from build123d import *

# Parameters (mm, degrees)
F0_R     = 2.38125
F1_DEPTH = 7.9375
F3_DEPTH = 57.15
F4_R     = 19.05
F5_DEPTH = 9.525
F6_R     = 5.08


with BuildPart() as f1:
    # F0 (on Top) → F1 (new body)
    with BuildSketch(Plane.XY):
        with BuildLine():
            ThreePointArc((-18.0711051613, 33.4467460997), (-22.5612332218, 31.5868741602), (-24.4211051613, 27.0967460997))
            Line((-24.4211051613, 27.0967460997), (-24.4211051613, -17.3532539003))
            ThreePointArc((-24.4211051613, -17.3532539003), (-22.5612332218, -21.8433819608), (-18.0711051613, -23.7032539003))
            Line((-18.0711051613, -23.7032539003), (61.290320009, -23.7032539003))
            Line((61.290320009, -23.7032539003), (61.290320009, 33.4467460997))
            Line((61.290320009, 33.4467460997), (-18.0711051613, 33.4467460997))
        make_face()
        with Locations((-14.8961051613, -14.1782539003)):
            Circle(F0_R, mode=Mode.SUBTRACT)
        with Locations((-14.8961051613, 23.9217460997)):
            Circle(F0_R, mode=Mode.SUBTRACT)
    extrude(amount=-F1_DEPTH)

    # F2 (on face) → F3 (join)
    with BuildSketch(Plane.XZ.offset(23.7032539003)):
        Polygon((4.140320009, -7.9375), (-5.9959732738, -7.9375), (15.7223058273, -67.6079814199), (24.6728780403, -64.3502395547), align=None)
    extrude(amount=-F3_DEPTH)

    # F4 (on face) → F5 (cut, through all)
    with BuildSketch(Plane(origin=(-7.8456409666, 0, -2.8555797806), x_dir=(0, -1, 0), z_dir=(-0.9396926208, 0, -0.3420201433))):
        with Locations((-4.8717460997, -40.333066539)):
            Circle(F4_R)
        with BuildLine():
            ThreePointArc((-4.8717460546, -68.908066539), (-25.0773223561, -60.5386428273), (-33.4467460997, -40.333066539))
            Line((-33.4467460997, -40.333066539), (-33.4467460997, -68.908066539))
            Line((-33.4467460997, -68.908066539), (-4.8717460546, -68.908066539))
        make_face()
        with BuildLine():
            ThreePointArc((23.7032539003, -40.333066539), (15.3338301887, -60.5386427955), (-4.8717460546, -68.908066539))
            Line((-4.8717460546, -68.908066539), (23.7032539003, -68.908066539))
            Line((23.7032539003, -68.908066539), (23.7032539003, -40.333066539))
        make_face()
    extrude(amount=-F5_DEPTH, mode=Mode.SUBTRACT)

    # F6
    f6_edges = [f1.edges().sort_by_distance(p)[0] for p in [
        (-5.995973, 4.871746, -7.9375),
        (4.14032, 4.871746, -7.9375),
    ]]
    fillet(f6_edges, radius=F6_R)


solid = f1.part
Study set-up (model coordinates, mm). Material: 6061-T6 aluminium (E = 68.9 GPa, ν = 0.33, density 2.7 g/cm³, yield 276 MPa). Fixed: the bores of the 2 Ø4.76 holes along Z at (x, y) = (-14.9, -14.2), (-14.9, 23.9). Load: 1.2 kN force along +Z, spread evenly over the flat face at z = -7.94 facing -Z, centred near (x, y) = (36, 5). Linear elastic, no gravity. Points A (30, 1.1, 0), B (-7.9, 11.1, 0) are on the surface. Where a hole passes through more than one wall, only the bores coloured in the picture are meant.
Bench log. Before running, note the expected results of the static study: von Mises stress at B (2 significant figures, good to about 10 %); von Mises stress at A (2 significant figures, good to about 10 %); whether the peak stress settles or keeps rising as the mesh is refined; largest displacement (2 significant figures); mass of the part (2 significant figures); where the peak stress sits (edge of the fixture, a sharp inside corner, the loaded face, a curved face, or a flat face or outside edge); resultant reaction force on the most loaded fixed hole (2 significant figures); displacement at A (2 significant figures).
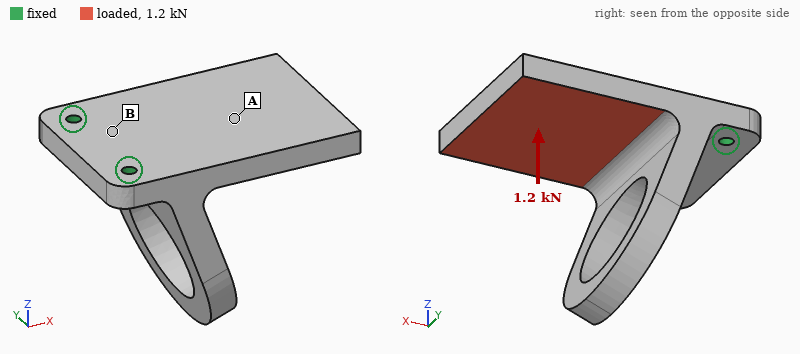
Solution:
53 MPa
18 MPa
keeps rising
0.51 mm
160 g
edge of the fixture
610 N
0.24 mm
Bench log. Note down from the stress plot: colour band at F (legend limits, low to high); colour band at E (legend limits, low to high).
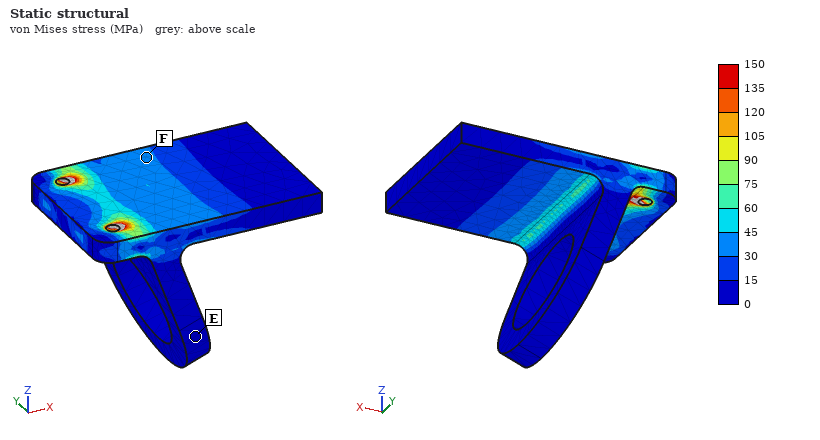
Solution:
30 to 45 MPa
0 to 15 MPa
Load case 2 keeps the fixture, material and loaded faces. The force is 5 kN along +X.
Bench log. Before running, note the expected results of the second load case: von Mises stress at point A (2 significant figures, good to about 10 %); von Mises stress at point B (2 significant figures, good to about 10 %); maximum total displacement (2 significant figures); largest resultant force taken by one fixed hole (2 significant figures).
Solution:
12 MPa
14 MPa
0.24 mm
2.5 kN
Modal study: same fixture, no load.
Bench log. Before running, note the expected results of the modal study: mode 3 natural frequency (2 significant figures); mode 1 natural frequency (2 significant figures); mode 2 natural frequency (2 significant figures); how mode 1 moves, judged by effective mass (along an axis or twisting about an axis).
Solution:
3300 Hz
1000 Hz
2300 Hz
along Z
